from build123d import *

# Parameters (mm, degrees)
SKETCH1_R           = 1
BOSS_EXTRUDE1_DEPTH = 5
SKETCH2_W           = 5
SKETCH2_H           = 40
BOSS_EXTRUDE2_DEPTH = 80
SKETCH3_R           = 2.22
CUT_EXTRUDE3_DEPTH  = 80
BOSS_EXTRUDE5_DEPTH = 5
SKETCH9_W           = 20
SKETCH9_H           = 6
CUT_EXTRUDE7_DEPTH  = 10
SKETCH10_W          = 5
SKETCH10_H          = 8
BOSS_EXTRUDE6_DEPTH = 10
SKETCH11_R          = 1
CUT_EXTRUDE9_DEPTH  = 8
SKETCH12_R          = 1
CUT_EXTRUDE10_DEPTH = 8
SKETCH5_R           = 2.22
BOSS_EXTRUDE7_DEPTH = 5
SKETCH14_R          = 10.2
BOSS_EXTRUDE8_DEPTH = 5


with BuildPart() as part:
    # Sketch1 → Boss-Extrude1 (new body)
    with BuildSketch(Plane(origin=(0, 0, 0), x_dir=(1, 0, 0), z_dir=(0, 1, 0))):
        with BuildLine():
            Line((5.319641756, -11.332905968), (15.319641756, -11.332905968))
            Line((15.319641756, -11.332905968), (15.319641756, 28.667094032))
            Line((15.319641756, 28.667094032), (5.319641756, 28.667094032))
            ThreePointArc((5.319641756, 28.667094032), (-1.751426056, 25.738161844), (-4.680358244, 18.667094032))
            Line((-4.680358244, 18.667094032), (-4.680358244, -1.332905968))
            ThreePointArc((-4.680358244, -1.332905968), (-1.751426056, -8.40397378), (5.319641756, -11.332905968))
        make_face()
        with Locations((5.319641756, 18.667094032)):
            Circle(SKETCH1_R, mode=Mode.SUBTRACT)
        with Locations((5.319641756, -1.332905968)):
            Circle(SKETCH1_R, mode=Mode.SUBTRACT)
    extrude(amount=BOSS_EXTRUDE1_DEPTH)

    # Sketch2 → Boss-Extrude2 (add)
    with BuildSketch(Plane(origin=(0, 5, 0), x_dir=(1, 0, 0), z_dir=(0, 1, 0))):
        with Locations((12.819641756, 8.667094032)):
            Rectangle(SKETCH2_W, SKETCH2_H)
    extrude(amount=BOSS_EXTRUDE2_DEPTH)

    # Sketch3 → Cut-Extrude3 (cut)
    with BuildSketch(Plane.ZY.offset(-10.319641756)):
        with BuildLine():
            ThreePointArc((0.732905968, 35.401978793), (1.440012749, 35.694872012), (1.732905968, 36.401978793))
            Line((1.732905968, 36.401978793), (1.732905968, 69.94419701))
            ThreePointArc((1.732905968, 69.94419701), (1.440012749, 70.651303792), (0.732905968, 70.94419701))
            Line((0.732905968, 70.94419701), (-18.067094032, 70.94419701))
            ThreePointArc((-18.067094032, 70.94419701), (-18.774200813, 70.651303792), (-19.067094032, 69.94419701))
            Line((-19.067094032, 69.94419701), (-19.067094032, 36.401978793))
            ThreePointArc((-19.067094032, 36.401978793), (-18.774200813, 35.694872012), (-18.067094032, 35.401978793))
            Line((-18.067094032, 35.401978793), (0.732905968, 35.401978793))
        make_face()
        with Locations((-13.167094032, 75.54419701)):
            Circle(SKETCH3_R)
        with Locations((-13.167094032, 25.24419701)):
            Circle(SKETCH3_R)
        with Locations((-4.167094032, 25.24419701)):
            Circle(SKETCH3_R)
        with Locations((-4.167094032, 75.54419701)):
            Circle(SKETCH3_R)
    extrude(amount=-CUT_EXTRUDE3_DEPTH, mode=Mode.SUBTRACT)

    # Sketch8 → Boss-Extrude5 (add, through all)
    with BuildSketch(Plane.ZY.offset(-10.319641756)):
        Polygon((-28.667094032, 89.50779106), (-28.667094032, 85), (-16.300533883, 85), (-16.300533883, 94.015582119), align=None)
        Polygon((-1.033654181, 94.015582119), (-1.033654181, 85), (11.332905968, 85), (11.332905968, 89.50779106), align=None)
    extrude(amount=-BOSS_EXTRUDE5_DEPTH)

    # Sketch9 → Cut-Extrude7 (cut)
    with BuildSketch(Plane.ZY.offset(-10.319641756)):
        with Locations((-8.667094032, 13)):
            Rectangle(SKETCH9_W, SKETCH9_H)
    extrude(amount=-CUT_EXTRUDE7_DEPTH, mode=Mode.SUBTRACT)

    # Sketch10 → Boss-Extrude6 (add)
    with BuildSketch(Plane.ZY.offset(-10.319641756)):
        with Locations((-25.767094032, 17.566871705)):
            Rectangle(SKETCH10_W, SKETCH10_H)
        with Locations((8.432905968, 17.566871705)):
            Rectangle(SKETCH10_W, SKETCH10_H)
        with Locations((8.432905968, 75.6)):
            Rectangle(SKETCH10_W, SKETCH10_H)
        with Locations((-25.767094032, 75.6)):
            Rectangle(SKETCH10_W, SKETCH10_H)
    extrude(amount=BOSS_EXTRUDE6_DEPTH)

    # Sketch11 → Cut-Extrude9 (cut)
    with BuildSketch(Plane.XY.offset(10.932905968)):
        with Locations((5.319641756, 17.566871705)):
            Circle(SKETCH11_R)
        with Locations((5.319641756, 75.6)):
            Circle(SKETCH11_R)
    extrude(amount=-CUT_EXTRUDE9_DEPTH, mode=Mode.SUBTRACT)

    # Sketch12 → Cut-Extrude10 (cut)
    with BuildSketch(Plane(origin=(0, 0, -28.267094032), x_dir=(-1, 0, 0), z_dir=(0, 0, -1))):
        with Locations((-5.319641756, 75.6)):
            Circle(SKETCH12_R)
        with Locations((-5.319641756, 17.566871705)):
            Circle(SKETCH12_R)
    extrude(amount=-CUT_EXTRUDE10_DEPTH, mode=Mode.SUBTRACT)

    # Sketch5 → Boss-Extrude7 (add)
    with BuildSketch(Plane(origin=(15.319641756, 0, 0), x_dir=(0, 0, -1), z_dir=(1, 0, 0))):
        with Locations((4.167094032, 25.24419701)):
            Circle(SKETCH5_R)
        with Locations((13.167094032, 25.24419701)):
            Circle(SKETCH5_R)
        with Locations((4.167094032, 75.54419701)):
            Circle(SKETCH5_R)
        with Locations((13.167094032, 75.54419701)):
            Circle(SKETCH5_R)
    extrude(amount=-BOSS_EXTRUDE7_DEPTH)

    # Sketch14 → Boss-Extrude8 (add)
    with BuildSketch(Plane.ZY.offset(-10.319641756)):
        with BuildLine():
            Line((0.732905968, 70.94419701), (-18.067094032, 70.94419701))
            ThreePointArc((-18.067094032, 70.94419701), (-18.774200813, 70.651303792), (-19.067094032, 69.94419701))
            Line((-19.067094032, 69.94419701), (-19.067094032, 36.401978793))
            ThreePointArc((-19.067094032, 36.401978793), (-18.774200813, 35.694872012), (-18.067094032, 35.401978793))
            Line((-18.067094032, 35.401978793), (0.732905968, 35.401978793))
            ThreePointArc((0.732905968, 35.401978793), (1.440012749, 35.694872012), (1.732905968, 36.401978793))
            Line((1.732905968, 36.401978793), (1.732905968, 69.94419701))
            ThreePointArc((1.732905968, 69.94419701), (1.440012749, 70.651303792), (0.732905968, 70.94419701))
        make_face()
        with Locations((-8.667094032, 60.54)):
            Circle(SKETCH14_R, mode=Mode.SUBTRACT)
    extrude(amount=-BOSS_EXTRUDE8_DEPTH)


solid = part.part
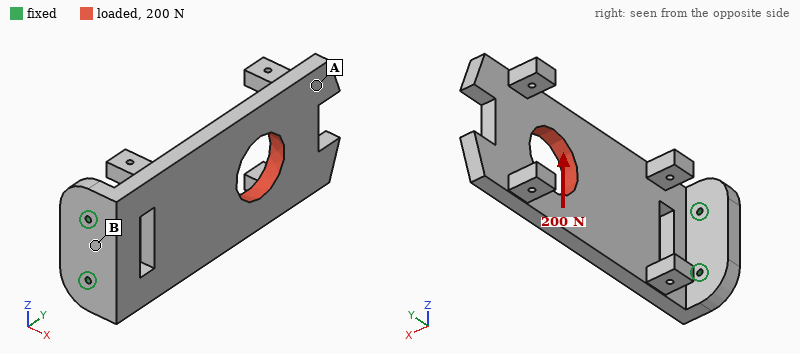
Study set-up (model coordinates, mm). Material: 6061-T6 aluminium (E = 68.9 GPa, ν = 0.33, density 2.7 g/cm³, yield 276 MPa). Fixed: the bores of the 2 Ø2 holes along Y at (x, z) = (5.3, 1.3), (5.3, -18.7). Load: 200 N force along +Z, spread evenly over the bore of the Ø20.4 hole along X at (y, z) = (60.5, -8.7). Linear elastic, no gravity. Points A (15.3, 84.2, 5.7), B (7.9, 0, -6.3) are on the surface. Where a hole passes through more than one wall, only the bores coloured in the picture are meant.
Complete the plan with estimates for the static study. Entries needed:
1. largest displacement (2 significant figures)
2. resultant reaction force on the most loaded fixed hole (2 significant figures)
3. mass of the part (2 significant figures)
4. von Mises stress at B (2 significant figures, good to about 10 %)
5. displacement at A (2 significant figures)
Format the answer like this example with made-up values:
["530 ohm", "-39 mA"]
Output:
["85 µm", "500 N", "54 g", "12 MPa", "74 µm"]
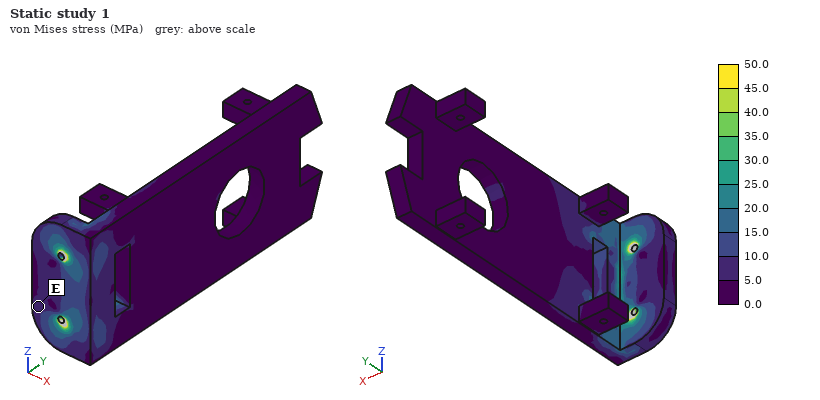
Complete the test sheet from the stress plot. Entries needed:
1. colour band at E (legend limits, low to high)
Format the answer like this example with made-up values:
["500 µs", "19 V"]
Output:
["5.0 to 10.0 MPa"]
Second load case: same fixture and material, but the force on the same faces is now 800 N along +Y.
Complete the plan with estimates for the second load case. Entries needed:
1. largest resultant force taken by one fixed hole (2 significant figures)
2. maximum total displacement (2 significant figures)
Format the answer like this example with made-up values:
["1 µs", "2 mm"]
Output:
["400 N", "0.14 mm"]
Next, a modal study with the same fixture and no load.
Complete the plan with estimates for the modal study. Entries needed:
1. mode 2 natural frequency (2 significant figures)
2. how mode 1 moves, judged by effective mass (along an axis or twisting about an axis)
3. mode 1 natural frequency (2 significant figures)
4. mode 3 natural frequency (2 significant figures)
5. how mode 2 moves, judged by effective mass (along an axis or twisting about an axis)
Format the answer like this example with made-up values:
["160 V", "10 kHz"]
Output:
["1500 Hz", "along X", "400 Hz", "2000 Hz", "along Z"]
